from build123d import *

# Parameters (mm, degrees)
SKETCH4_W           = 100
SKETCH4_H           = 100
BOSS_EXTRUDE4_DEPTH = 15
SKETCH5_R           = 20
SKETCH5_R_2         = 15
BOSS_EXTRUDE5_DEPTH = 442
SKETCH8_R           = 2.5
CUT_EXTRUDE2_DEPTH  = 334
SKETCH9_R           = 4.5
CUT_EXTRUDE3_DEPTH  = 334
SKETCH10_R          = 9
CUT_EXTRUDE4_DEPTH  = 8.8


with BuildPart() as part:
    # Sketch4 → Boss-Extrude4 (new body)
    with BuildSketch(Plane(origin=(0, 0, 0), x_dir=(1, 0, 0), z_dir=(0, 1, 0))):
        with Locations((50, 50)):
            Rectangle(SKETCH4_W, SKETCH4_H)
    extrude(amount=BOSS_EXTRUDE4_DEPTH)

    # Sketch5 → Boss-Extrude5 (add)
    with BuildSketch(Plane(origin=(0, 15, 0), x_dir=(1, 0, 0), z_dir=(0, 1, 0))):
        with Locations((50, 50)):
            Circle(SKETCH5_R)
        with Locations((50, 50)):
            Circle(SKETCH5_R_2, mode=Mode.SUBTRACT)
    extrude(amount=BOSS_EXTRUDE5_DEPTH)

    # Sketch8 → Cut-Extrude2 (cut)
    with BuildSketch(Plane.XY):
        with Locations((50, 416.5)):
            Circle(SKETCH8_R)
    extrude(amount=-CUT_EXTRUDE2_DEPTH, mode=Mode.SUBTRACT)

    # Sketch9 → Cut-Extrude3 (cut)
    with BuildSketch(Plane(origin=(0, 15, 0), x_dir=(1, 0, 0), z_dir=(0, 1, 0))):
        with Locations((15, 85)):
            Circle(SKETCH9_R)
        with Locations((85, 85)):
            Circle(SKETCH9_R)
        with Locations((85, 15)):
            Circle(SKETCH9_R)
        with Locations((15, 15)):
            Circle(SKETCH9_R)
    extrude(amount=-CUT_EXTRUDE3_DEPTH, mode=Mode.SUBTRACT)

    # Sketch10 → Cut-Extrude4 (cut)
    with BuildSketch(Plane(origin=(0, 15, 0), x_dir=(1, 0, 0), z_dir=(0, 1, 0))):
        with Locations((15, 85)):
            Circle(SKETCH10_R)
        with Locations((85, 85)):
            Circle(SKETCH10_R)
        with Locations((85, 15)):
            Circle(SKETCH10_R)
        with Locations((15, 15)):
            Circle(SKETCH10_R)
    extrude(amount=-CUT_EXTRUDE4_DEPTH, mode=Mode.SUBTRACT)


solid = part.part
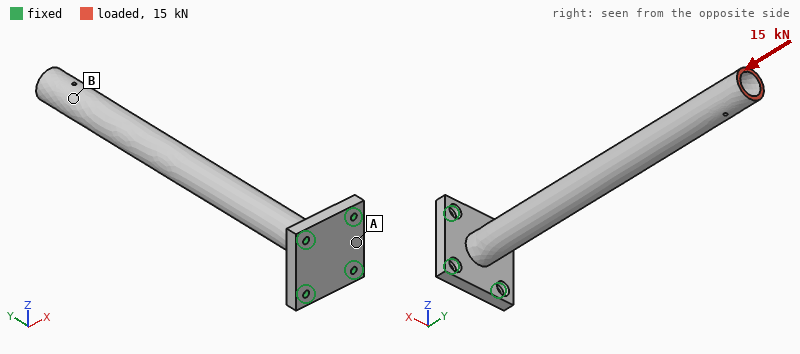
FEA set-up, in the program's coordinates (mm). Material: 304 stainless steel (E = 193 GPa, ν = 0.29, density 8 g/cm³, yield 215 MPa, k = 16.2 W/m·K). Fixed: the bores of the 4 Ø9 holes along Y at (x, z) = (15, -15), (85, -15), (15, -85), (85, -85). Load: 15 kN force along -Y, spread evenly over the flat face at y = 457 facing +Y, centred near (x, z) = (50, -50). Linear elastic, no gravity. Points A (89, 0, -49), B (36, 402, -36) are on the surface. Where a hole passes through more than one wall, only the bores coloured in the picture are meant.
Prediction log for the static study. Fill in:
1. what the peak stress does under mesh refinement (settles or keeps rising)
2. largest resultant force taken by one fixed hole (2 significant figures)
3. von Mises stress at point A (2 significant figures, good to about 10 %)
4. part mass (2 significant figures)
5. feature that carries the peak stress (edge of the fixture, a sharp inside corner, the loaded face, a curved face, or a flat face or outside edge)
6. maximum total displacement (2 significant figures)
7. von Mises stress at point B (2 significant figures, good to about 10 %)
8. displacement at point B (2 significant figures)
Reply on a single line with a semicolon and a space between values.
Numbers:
keeps rising; 5.2 kN; 18 MPa; 3.1 kg; edge of the fixture; 77 µm; 28 MPa; 69 µm
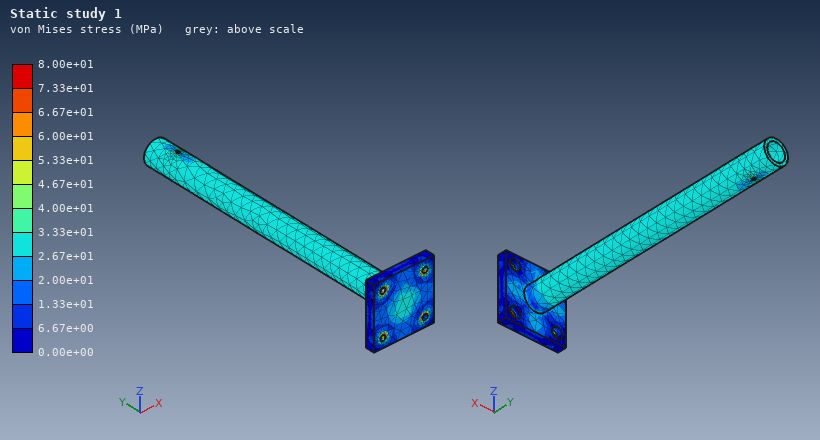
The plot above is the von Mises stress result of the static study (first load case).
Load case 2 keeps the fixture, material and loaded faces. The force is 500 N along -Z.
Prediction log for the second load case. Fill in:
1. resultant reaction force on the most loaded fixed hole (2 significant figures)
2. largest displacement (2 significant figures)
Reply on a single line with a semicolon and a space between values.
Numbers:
2.0 kN; 1.0 mm
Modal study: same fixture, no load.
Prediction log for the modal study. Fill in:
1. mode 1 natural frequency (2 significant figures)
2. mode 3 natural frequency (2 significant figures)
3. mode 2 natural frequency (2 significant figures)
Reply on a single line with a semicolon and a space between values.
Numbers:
160 Hz; 960 Hz; 160 Hz
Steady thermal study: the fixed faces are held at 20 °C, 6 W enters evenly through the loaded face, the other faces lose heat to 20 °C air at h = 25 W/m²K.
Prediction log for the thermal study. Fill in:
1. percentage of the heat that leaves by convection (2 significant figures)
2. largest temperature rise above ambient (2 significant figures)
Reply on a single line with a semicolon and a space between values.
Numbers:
100 %; 27 K
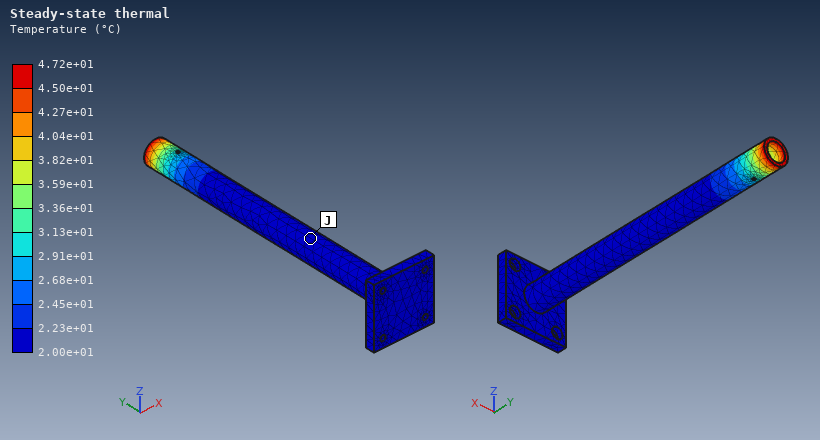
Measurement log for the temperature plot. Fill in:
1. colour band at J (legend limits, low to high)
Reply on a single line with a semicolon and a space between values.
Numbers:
2.00e+01 to 2.23e+01 °C
